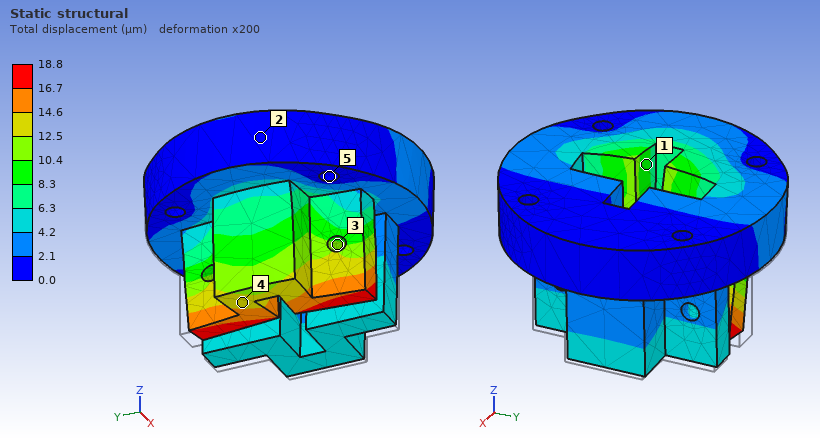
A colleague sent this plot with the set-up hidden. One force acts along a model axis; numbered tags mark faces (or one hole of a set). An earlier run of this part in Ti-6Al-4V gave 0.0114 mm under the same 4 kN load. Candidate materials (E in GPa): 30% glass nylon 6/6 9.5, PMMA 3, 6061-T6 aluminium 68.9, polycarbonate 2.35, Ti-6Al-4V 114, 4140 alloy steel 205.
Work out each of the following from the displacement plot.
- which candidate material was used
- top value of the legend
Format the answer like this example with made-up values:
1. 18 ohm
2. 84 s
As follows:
1. 6061-T6 aluminium
2. 18.8 µm
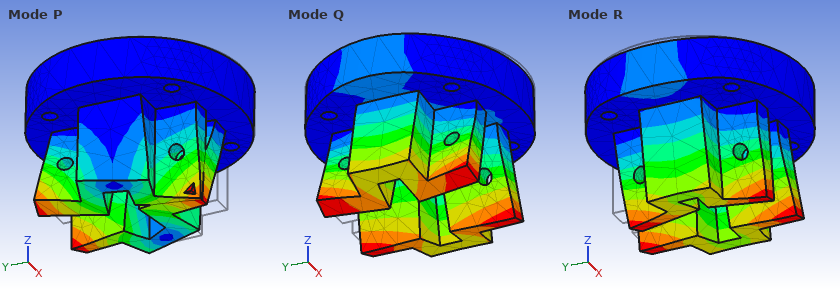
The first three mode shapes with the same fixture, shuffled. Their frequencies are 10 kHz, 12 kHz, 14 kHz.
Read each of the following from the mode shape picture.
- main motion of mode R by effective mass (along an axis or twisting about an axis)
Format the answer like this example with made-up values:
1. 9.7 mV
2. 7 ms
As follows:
1. along X
